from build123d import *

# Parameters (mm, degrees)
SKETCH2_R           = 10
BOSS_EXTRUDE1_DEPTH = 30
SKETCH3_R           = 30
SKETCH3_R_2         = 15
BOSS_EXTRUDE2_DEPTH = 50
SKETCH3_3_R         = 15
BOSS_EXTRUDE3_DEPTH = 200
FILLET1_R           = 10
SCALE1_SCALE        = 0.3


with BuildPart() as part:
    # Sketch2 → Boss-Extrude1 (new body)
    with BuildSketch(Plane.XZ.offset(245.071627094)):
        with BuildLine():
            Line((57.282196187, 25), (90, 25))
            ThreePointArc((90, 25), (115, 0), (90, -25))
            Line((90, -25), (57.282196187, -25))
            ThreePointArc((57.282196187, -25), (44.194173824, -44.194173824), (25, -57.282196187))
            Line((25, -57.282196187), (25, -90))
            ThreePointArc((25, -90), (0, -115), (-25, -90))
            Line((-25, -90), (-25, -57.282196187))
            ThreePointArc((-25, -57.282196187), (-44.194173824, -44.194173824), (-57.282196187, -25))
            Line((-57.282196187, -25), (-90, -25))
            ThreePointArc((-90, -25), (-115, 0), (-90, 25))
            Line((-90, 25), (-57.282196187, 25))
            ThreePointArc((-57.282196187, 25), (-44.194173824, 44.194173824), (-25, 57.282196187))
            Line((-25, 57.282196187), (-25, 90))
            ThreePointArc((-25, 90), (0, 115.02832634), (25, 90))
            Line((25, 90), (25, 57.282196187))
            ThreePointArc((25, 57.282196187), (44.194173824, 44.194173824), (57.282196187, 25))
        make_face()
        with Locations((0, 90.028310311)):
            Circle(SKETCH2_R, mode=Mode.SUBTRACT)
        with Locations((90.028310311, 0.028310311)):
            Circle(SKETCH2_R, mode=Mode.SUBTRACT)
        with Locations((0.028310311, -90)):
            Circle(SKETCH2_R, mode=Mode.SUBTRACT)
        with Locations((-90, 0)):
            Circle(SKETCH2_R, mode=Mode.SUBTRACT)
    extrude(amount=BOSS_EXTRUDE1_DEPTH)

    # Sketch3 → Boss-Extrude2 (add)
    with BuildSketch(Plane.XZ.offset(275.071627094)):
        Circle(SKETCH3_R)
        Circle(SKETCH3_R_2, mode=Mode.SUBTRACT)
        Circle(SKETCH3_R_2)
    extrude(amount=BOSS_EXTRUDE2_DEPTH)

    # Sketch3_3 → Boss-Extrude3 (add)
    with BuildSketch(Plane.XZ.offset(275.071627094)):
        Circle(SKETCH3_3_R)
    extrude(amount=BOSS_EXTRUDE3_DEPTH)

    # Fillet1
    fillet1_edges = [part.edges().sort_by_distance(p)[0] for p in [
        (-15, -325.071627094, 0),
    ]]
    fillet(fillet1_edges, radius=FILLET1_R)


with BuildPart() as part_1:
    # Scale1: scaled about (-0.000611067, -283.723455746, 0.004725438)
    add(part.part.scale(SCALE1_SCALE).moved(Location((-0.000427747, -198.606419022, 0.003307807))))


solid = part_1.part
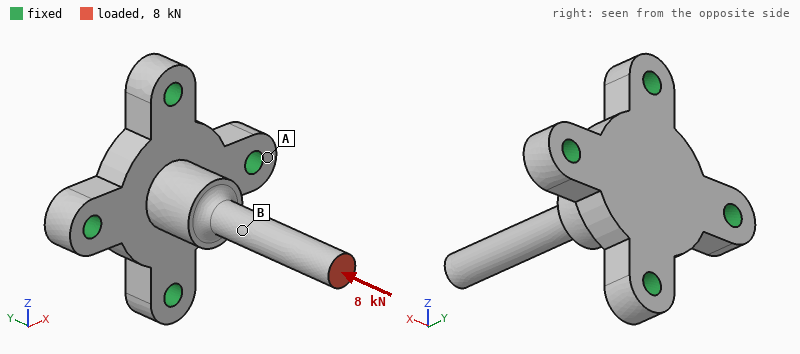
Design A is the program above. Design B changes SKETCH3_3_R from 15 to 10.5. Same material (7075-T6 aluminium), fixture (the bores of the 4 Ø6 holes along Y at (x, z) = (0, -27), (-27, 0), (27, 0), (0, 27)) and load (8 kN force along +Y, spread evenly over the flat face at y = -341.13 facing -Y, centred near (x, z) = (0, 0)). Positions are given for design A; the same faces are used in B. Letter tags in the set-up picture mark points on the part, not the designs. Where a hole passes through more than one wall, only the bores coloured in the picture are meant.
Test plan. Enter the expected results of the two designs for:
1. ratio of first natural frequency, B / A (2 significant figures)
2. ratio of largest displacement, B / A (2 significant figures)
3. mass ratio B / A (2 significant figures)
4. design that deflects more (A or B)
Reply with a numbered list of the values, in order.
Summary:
1. 0.78
2. 1.7
3. 0.94
4. B
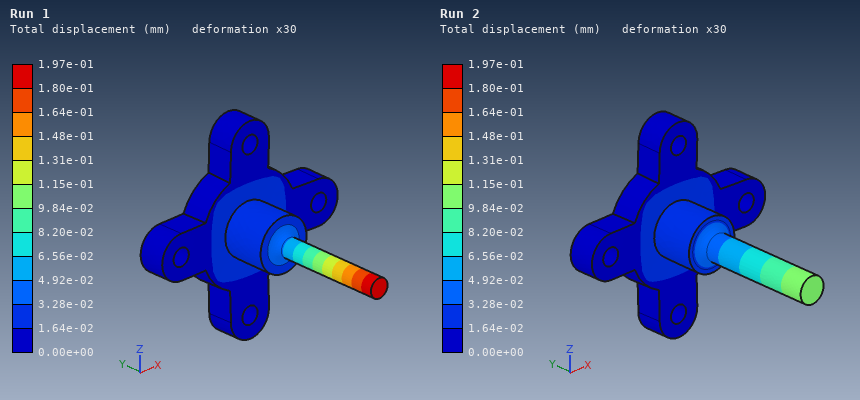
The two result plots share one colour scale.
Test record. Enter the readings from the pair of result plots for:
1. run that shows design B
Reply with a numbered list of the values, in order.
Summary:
1. Run 1
